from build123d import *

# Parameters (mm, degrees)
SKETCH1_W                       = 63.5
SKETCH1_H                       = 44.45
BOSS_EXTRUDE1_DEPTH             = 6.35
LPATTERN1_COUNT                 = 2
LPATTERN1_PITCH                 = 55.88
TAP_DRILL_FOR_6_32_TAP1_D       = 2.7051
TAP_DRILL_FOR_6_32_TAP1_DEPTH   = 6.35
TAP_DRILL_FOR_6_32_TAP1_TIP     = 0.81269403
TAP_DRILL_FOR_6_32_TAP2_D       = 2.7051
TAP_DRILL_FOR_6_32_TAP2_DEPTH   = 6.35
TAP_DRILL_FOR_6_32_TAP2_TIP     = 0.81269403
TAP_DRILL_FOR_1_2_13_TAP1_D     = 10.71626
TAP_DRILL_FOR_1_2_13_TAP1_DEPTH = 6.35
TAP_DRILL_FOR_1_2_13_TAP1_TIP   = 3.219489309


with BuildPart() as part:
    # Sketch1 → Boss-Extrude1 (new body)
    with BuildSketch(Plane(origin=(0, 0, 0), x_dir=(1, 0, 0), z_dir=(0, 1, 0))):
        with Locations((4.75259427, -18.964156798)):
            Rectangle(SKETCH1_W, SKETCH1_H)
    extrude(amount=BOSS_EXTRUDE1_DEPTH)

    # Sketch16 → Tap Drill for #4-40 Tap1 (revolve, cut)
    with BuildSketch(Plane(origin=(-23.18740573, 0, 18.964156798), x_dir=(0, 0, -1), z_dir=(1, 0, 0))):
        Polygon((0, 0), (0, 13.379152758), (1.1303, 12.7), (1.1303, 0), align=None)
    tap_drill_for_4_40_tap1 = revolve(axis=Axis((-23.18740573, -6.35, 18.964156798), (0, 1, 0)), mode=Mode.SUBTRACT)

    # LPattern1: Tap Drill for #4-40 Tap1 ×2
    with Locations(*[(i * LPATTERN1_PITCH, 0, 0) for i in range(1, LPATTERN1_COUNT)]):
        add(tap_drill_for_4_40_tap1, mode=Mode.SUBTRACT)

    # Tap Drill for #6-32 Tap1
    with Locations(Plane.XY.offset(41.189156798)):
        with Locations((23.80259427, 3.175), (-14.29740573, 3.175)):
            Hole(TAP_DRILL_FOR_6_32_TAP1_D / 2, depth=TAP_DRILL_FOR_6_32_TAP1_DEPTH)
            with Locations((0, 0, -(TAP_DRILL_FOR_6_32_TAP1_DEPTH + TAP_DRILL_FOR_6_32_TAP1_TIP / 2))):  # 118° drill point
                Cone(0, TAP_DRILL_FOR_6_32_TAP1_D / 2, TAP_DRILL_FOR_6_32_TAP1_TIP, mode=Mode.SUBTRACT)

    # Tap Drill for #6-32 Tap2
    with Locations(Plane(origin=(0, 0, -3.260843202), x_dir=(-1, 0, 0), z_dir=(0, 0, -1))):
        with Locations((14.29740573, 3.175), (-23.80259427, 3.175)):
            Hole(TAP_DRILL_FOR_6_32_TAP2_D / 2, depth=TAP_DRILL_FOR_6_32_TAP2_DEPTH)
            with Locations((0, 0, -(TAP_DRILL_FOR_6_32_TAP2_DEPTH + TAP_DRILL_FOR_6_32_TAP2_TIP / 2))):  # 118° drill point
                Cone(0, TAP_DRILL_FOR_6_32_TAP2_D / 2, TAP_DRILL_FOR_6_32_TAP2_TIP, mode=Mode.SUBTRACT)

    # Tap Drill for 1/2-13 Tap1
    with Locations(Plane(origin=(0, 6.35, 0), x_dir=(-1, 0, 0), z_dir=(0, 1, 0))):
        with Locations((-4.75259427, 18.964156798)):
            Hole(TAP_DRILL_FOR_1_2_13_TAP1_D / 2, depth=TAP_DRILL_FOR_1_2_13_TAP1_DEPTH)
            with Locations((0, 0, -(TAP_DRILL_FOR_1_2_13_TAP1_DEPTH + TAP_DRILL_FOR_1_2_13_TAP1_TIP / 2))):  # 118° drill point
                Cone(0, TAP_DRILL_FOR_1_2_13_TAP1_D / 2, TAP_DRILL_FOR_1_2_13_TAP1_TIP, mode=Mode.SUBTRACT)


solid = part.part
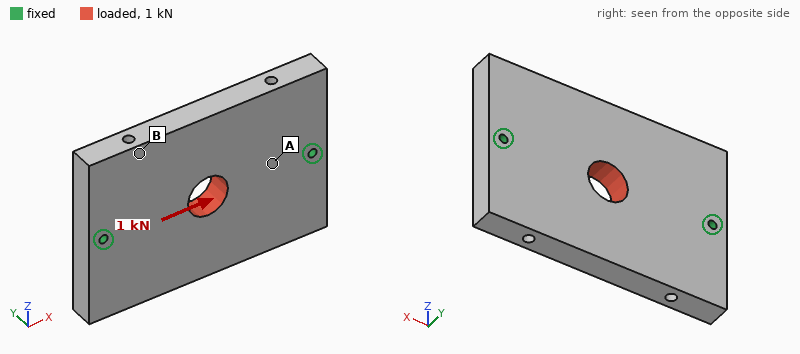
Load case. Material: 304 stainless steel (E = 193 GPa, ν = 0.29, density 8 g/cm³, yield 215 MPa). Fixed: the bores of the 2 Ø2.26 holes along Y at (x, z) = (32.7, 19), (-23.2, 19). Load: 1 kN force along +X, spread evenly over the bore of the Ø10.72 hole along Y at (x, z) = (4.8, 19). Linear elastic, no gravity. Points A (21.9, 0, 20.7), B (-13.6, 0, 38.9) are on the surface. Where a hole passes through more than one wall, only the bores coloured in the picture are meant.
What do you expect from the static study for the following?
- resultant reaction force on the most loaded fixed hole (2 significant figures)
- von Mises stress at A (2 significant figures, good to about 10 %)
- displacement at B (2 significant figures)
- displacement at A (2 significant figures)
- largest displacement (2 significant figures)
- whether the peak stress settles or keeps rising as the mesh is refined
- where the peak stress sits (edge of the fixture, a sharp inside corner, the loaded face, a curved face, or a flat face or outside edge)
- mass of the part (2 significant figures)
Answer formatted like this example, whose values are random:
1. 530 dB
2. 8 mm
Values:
1. 500 N
2. 5.3 MPa
3. 0.51 µm
4. 0.40 µm
5. 0.75 µm
6. keeps rising
7. edge of the fixture
8. 140 g
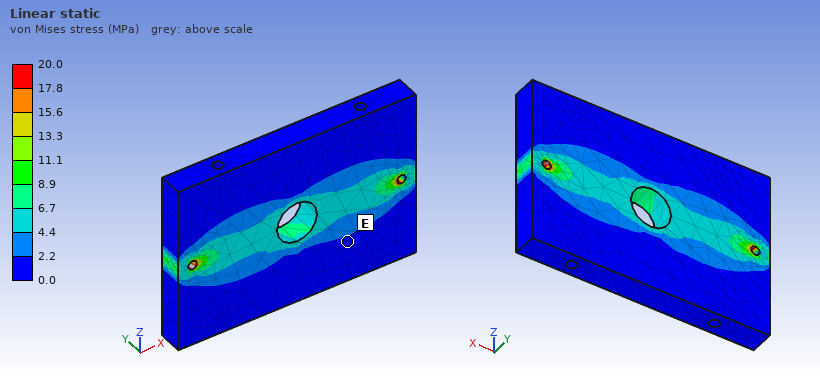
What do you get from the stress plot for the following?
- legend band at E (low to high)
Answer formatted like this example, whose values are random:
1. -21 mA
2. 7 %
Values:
1. 0.0 to 2.2 MPa
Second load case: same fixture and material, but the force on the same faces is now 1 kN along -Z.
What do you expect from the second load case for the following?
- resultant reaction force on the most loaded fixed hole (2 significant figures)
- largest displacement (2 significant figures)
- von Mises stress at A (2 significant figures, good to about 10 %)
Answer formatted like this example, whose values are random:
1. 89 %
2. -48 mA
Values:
1. 500 N
2. 1.3 µm
3. 3.8 MPa
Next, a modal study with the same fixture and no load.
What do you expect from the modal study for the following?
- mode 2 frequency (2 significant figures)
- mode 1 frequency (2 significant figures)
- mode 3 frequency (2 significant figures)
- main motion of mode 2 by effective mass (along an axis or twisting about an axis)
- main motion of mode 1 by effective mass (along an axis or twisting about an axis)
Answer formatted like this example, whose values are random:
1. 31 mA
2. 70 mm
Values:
1. 5700 Hz
2. 4500 Hz
3. 9700 Hz
4. along Y
5. twisting about X
